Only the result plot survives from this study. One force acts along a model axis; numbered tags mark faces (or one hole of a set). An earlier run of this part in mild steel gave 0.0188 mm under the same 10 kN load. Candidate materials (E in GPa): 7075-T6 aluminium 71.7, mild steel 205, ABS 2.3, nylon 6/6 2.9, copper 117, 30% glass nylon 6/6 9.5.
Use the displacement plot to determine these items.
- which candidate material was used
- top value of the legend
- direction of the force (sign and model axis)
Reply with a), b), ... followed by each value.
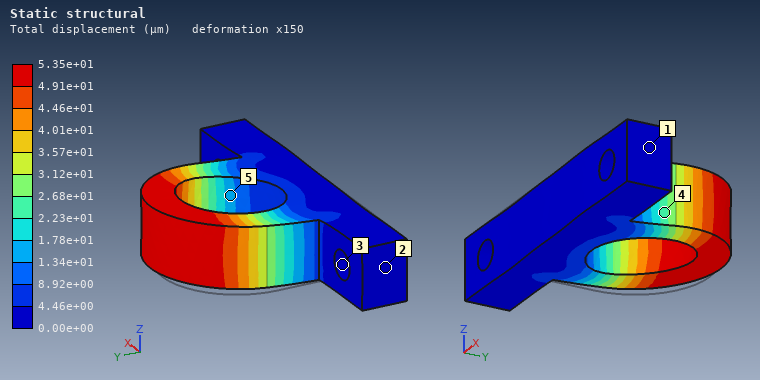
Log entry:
a) 7075-T6 aluminium
b) 5.35e+01 µm
c) +X
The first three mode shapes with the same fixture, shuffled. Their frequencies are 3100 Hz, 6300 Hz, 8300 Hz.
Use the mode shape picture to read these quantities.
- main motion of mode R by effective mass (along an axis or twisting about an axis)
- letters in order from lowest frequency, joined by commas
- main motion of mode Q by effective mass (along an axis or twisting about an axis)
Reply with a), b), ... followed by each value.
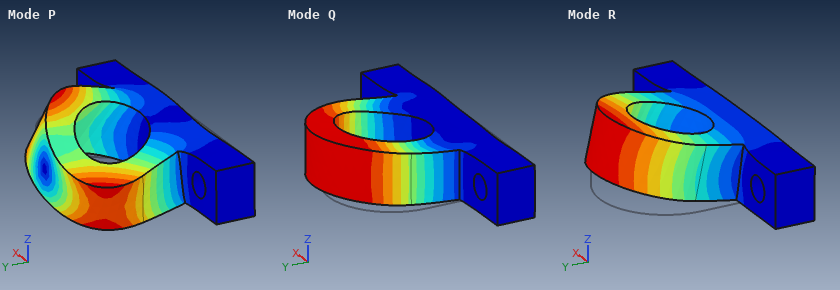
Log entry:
a) along Z
b) R, Q, P
c) along X
